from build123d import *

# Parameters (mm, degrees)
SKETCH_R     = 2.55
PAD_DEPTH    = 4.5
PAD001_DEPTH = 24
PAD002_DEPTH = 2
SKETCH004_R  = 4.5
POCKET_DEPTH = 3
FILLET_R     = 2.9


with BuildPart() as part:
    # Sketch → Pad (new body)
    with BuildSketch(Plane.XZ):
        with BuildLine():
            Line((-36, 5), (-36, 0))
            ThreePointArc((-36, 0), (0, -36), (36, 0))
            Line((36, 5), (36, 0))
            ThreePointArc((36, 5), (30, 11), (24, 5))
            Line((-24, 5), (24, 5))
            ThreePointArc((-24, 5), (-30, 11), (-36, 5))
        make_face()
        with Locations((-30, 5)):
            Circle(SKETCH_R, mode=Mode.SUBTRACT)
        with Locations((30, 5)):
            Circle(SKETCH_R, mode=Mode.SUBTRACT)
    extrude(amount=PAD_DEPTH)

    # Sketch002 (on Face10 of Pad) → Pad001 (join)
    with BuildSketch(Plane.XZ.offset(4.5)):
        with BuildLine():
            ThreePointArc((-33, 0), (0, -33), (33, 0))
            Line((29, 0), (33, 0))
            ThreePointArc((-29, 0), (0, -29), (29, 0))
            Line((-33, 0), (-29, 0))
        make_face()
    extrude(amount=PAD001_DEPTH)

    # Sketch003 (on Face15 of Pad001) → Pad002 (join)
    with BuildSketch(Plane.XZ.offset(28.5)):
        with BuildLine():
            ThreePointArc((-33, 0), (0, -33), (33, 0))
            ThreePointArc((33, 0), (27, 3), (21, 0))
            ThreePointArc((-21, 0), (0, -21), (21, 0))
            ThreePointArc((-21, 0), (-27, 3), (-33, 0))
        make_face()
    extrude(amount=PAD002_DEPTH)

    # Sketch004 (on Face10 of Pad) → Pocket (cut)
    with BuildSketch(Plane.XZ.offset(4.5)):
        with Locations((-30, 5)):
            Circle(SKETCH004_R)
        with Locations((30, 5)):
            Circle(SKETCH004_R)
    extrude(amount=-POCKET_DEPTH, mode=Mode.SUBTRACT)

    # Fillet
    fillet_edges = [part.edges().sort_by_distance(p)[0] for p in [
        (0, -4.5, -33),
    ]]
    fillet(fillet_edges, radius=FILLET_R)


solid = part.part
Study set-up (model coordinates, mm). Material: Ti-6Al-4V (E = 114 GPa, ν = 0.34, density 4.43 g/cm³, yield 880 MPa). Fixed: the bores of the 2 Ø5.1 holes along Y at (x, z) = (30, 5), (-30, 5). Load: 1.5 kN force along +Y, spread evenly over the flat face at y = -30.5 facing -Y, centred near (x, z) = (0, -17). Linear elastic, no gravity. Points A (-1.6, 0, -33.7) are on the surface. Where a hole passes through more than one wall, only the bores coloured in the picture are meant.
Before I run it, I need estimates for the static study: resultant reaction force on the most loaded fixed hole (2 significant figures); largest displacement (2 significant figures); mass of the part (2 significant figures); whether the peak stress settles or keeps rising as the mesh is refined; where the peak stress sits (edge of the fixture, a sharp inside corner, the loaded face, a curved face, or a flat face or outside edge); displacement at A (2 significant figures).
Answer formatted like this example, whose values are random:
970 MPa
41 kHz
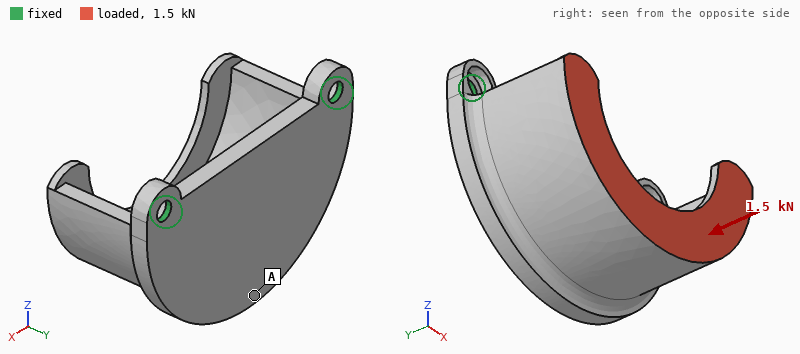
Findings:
750 N
1.1 mm
100 g
keeps rising
edge of the fixture
0.84 mm
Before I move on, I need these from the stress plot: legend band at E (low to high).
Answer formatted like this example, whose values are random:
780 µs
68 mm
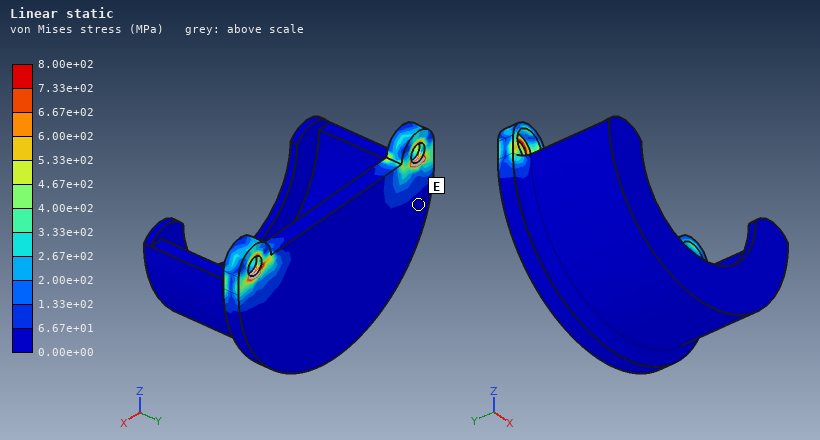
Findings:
0.00e+00 to 6.67e+01 MPa
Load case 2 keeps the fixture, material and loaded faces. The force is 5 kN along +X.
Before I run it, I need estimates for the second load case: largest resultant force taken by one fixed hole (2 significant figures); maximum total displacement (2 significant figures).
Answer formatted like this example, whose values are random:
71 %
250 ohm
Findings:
3.7 kN
0.94 mm
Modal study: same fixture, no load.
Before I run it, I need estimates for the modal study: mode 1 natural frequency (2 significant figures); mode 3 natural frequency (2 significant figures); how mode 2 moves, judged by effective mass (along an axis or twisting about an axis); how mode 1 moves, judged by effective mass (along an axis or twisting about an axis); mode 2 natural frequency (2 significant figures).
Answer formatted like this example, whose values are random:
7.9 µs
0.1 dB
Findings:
690 Hz
6400 Hz
along X
along Y
2600 Hz
